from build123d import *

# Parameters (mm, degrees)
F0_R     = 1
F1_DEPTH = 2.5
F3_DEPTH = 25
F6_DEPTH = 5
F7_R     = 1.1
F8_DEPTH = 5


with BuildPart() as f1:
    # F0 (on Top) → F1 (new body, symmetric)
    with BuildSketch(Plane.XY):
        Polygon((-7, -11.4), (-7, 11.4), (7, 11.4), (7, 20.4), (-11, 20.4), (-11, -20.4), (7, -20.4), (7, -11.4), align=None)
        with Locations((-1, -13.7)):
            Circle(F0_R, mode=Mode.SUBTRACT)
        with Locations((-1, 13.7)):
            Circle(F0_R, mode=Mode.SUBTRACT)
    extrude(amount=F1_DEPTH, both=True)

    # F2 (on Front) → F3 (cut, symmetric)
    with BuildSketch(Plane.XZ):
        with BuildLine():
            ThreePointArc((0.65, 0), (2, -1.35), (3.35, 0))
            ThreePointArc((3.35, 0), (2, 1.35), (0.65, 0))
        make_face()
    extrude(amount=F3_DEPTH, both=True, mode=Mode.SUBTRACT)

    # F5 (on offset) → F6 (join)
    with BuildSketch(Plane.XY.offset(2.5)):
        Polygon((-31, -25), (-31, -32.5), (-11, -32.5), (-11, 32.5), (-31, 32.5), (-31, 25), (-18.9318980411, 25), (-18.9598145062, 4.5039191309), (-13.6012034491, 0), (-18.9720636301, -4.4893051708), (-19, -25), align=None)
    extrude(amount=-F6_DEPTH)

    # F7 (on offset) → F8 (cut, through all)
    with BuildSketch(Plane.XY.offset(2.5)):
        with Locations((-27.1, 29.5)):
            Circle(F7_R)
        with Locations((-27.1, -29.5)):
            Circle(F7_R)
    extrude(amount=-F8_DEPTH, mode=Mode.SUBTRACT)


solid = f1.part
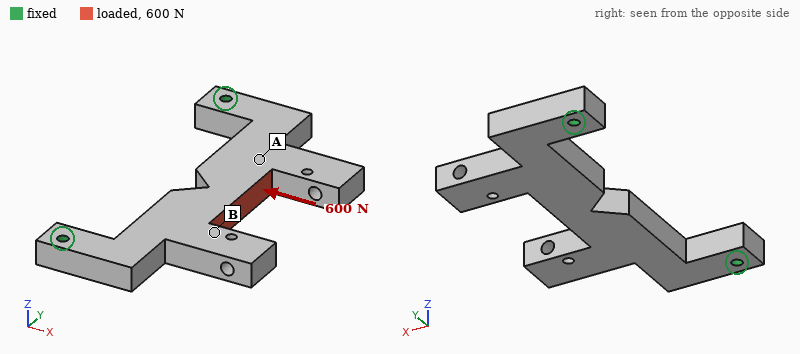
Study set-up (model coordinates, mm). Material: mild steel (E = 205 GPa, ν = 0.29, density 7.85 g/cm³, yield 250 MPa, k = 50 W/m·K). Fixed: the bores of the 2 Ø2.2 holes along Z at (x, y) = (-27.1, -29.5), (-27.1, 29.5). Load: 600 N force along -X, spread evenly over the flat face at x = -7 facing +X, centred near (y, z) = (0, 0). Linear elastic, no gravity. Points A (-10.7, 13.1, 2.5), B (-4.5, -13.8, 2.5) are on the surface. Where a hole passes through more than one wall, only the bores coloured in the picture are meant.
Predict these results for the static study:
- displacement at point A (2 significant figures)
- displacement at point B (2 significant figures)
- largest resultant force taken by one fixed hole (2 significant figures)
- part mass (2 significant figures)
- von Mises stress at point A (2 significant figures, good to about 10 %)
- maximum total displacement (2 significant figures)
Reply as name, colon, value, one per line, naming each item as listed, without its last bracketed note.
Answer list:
displacement at point A: 6.6 µm
displacement at point B: 7.1 µm
largest resultant force taken by one fixed hole: 450 N
part mass: 41 g
von Mises stress at point A: 15 MPa
maximum total displacement: 12 µm
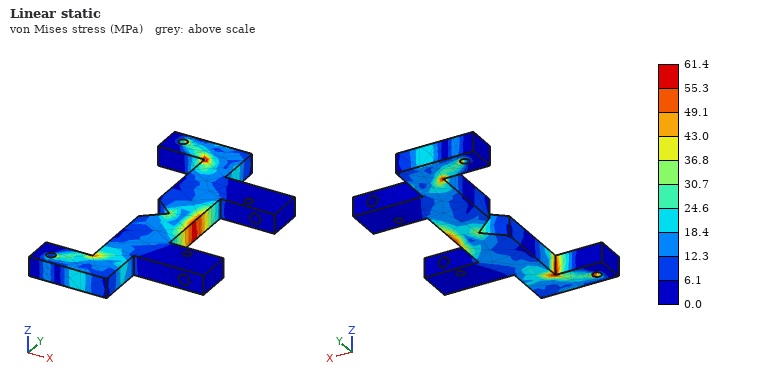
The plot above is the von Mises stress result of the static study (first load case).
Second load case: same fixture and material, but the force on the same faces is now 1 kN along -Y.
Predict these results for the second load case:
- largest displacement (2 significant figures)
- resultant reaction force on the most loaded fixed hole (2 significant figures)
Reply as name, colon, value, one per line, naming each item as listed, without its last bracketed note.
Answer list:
largest displacement: 8.2 µm
resultant reaction force on the most loaded fixed hole: 560 N
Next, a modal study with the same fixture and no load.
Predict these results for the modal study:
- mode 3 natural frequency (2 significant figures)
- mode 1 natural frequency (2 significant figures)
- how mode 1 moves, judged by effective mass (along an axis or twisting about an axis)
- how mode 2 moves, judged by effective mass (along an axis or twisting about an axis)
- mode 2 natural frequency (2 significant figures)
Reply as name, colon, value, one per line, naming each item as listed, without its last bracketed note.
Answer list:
mode 3 natural frequency: 6800 Hz
mode 1 natural frequency: 2500 Hz
how mode 1 moves, judged by effective mass: along Z
how mode 2 moves, judged by effective mass: twisting about X
mode 2 natural frequency: 5300 Hz
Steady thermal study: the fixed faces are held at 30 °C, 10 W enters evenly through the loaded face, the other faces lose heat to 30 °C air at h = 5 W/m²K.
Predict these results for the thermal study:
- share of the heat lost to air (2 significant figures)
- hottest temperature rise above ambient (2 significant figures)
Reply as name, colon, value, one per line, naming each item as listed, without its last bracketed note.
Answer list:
share of the heat lost to air: 7.3 %
hottest temperature rise above ambient: 73 K
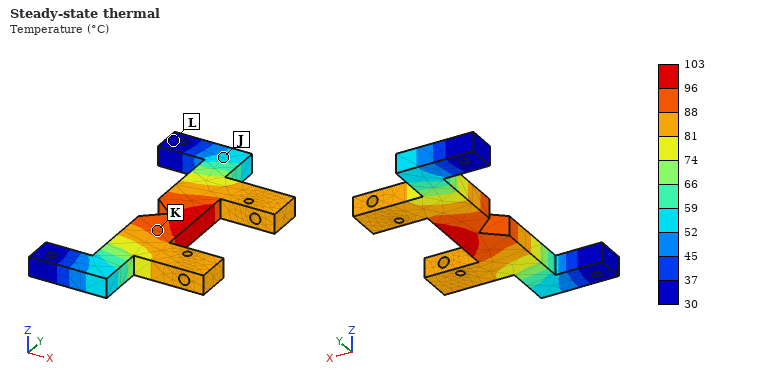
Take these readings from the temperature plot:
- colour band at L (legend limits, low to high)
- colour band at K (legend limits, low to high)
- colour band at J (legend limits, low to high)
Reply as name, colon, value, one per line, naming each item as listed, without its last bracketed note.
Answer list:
colour band at L: 30 to 37 °C
colour band at K: 88 to 96 °C
colour band at J: 52 to 59 °C
